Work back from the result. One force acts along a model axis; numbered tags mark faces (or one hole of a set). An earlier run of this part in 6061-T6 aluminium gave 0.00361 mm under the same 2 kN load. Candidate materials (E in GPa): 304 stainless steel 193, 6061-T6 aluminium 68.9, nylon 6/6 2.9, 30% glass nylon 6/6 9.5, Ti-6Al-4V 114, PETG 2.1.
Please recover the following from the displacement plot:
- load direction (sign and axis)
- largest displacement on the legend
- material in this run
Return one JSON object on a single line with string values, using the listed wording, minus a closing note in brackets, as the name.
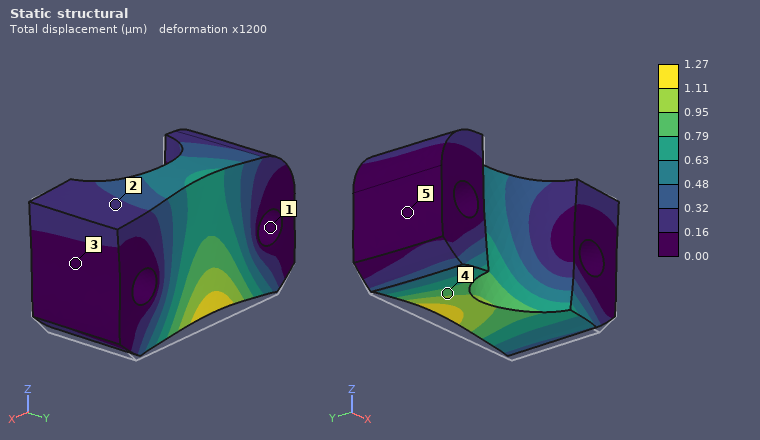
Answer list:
{"load direction": "+Z", "largest displacement on the legend": "1.27 µm", "material in this run": "304 stainless steel"}
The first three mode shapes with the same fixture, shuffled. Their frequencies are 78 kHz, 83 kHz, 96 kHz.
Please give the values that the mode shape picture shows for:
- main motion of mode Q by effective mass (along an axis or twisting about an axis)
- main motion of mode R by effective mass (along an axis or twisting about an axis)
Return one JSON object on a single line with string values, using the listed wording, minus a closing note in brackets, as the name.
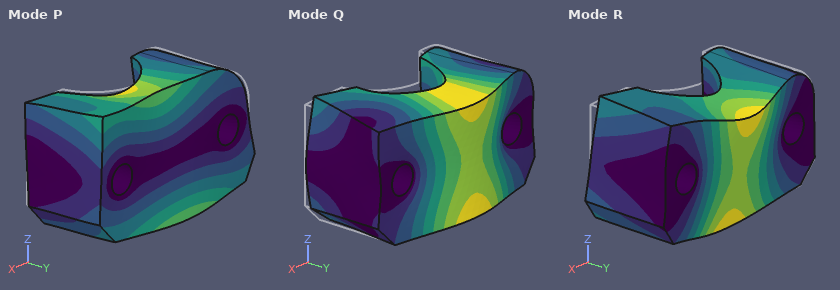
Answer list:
{"main motion of mode Q by effective mass": "along Y", "main motion of mode R by effective mass": "along Z"}
